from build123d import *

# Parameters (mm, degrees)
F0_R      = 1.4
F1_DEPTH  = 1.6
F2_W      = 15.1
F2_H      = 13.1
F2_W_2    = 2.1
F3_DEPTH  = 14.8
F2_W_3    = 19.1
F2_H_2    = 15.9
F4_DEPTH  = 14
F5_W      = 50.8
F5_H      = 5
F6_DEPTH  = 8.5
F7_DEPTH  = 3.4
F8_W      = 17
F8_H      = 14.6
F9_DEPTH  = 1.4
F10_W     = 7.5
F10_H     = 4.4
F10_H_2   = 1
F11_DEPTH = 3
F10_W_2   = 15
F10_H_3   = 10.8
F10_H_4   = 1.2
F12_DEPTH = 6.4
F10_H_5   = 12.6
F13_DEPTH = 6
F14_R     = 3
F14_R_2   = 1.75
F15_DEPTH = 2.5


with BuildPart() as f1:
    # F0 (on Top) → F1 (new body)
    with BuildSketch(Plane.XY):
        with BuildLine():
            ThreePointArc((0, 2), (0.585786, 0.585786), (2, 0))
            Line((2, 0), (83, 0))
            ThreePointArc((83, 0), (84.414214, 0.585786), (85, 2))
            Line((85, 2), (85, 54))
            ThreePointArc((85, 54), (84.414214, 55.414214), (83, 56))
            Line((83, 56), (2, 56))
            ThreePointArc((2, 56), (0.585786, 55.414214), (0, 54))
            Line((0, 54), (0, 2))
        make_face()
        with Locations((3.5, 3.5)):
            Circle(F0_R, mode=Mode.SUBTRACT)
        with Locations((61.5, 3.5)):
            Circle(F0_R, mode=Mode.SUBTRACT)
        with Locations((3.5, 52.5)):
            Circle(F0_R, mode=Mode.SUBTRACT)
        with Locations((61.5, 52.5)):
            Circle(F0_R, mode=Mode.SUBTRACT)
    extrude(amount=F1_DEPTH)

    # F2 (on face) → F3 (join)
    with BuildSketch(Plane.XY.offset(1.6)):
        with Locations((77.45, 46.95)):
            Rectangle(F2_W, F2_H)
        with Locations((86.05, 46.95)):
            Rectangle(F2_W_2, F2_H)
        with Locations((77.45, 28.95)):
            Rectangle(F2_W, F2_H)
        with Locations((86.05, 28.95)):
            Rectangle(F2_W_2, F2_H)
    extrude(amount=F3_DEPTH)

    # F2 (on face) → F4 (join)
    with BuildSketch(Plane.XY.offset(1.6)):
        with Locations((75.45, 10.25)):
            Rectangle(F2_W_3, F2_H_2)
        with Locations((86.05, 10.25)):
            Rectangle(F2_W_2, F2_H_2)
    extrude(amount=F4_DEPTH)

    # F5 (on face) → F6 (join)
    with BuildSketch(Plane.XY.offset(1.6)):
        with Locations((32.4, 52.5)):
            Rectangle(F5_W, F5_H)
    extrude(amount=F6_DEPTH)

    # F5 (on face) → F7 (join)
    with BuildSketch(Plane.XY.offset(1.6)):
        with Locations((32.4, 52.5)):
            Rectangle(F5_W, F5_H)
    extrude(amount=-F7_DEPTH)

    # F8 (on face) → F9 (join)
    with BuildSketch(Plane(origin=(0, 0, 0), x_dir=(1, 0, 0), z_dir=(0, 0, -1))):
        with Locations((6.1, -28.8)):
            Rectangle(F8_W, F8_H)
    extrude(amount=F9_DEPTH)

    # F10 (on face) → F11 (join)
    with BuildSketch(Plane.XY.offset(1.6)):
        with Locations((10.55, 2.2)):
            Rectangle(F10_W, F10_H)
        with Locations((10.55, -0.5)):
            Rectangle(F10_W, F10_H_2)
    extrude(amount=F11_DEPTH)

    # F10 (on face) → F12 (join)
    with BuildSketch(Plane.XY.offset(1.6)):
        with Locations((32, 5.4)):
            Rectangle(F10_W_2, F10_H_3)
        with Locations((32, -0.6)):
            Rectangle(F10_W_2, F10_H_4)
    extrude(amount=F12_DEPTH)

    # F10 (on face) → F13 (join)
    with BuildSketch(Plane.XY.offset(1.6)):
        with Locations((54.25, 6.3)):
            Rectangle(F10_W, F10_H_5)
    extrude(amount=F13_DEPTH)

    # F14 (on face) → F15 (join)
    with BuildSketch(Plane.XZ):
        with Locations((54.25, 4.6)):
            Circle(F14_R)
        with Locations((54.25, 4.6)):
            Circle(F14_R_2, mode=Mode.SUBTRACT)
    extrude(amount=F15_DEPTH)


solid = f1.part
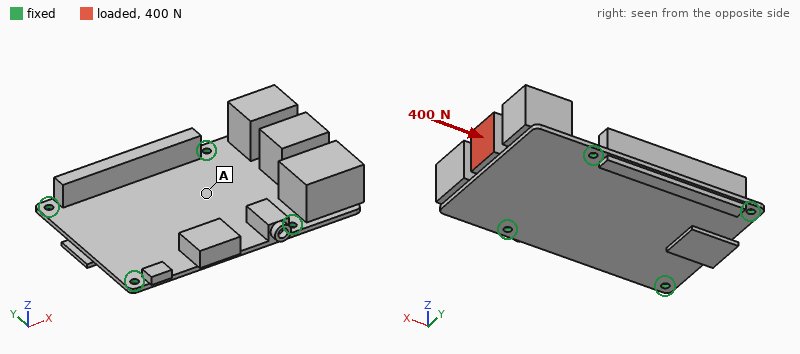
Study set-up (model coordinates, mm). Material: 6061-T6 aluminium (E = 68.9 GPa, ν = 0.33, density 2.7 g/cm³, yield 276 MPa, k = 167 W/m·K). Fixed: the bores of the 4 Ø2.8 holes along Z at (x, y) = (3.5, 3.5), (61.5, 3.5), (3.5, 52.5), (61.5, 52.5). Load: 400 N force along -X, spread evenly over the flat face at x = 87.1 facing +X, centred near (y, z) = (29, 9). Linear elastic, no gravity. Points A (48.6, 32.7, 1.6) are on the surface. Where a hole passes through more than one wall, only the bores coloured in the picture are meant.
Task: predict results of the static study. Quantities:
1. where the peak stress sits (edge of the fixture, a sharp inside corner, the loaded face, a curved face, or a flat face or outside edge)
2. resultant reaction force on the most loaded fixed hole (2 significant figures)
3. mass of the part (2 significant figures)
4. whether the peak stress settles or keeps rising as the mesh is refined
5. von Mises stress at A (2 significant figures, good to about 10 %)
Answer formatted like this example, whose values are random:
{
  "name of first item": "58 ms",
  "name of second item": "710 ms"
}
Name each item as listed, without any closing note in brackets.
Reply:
{
  "where the peak stress sits": "edge of the fixture",
  "resultant reaction force on the most loaded fixed hole": "150 N",
  "mass of the part": "64 g",
  "whether the peak stress settles or keeps rising as the mesh is refined": "keeps rising",
  "von Mises stress at A": "24 MPa"
}
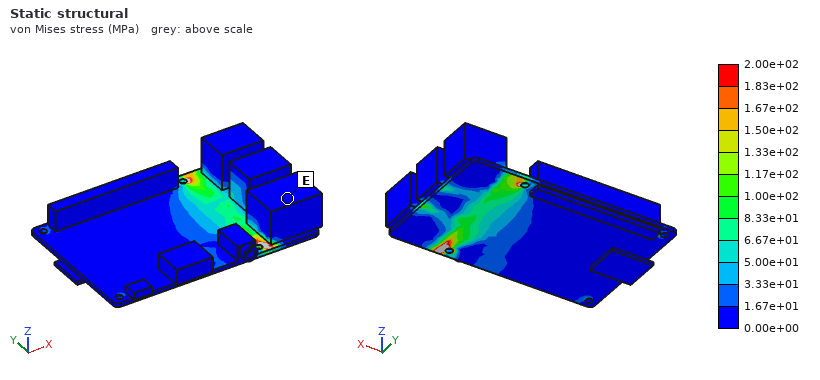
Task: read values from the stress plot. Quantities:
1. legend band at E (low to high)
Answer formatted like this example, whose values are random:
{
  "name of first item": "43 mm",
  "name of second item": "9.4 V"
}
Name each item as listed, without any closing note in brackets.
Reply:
{
  "legend band at E": "0.00e+00 to 1.67e+01 MPa"
}
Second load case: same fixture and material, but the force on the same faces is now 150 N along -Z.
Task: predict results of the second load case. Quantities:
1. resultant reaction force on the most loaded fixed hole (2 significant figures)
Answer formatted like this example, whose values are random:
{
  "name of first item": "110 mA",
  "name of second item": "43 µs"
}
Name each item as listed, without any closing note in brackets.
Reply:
{
  "resultant reaction force on the most loaded fixed hole": "93 N"
}
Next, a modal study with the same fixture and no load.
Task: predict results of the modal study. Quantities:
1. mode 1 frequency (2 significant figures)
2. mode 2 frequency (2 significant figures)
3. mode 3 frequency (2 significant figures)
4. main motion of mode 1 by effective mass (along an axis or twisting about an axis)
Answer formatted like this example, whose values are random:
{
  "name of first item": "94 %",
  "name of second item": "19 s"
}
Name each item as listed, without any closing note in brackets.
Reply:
{
  "mode 1 frequency": "590 Hz",
  "mode 2 frequency": "1900 Hz",
  "mode 3 frequency": "2100 Hz",
  "main motion of mode 1 by effective mass": "along Z"
}
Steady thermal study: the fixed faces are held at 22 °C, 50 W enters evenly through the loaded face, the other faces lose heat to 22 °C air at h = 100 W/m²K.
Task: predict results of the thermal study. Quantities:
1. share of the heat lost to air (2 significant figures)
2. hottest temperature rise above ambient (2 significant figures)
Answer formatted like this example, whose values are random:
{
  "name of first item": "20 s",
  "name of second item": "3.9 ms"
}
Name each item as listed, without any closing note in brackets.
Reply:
{
  "share of the heat lost to air": "49 %",
  "hottest temperature rise above ambient": "74 K"
}
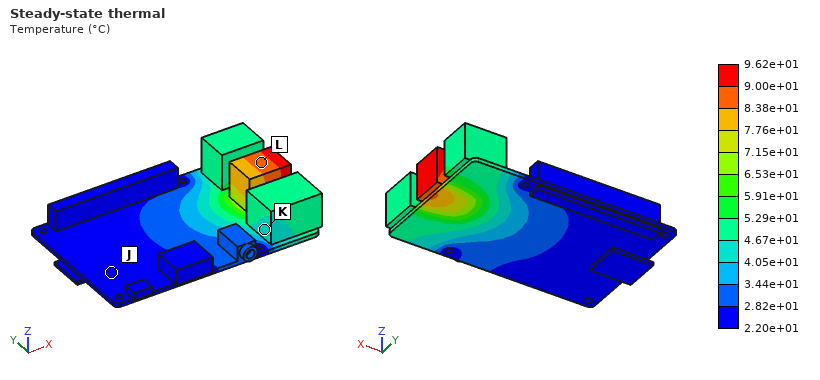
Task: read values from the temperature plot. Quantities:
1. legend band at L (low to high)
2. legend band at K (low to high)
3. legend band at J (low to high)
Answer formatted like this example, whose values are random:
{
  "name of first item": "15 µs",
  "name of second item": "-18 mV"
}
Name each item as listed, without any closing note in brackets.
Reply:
{
  "legend band at L": "8.38e+01 to 9.00e+01 °C",
  "legend band at K": "4.05e+01 to 4.67e+01 °C",
  "legend band at J": "2.20e+01 to 2.82e+01 °C"
}
